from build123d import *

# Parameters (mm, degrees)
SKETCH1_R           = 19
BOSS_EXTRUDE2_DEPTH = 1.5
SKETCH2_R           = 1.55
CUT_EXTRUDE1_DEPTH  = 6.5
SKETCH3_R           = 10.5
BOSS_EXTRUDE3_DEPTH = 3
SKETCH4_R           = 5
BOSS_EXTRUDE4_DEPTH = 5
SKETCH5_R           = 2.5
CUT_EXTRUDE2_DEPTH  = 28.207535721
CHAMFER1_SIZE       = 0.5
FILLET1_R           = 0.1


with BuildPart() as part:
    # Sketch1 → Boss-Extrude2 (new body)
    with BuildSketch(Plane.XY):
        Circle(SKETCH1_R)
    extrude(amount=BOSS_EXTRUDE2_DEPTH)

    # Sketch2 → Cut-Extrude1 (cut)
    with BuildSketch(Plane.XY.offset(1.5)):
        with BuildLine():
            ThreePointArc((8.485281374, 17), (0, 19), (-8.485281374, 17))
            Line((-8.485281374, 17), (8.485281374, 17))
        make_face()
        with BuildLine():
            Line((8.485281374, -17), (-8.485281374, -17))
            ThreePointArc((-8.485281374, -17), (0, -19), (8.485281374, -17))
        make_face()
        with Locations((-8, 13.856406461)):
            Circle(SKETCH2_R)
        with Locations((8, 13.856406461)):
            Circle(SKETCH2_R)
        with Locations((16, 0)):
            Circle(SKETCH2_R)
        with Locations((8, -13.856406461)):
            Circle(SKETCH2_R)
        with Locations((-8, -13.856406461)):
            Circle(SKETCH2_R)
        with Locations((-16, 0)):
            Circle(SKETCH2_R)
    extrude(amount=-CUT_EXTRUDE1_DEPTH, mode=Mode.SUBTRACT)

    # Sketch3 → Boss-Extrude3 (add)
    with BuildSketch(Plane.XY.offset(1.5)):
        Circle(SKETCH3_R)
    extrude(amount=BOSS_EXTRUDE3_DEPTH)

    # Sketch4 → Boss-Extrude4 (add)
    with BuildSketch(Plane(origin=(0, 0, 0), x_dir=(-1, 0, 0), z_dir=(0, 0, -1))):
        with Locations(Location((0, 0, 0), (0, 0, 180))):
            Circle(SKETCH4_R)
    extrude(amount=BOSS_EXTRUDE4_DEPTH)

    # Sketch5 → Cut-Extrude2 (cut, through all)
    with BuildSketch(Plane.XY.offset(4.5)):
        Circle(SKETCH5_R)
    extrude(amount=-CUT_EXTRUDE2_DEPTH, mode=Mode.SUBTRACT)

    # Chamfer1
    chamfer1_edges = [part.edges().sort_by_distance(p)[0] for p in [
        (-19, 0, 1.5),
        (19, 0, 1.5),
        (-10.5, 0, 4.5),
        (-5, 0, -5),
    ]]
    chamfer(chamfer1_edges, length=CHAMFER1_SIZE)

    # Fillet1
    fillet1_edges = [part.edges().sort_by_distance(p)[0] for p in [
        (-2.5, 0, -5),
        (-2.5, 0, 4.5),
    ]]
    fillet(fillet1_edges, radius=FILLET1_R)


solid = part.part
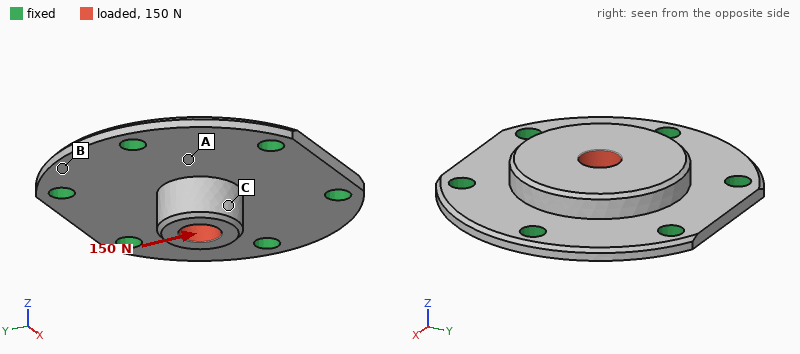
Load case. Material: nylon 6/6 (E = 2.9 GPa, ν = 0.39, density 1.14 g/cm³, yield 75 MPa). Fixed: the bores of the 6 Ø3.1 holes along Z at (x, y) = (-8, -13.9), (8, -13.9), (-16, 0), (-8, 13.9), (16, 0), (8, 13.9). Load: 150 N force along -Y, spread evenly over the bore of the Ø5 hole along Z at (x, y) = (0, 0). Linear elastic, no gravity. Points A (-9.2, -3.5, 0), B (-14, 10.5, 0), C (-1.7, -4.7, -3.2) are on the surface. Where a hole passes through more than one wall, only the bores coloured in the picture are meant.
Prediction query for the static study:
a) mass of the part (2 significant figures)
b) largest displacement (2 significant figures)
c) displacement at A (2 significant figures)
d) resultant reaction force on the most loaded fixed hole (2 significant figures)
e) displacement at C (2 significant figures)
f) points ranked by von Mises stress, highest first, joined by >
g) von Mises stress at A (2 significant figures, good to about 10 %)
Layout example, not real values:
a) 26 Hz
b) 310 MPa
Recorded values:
a) 3.2 g
b) 30 µm
c) 6.8 µm
d) 33 N
e) 25 µm
f) A > C > B
g) 1.8 MPa
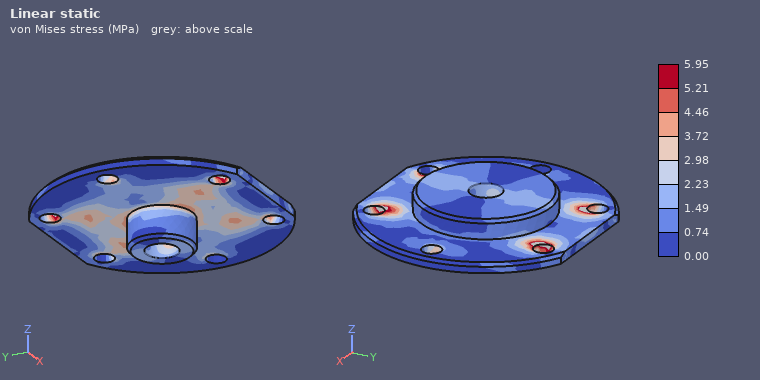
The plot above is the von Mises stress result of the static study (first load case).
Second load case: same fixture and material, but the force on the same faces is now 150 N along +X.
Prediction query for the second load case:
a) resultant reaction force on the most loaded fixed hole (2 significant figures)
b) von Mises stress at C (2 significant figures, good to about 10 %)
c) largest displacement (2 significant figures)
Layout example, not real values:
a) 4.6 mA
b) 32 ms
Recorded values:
a) 36 N
b) 0.84 MPa
c) 30 µm
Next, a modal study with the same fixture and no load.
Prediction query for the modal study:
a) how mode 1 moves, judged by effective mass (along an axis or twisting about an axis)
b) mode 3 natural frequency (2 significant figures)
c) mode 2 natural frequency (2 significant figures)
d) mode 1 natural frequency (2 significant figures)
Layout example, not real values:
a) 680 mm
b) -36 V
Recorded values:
a) along Z
b) 8700 Hz
c) 8700 Hz
d) 5300 Hz
